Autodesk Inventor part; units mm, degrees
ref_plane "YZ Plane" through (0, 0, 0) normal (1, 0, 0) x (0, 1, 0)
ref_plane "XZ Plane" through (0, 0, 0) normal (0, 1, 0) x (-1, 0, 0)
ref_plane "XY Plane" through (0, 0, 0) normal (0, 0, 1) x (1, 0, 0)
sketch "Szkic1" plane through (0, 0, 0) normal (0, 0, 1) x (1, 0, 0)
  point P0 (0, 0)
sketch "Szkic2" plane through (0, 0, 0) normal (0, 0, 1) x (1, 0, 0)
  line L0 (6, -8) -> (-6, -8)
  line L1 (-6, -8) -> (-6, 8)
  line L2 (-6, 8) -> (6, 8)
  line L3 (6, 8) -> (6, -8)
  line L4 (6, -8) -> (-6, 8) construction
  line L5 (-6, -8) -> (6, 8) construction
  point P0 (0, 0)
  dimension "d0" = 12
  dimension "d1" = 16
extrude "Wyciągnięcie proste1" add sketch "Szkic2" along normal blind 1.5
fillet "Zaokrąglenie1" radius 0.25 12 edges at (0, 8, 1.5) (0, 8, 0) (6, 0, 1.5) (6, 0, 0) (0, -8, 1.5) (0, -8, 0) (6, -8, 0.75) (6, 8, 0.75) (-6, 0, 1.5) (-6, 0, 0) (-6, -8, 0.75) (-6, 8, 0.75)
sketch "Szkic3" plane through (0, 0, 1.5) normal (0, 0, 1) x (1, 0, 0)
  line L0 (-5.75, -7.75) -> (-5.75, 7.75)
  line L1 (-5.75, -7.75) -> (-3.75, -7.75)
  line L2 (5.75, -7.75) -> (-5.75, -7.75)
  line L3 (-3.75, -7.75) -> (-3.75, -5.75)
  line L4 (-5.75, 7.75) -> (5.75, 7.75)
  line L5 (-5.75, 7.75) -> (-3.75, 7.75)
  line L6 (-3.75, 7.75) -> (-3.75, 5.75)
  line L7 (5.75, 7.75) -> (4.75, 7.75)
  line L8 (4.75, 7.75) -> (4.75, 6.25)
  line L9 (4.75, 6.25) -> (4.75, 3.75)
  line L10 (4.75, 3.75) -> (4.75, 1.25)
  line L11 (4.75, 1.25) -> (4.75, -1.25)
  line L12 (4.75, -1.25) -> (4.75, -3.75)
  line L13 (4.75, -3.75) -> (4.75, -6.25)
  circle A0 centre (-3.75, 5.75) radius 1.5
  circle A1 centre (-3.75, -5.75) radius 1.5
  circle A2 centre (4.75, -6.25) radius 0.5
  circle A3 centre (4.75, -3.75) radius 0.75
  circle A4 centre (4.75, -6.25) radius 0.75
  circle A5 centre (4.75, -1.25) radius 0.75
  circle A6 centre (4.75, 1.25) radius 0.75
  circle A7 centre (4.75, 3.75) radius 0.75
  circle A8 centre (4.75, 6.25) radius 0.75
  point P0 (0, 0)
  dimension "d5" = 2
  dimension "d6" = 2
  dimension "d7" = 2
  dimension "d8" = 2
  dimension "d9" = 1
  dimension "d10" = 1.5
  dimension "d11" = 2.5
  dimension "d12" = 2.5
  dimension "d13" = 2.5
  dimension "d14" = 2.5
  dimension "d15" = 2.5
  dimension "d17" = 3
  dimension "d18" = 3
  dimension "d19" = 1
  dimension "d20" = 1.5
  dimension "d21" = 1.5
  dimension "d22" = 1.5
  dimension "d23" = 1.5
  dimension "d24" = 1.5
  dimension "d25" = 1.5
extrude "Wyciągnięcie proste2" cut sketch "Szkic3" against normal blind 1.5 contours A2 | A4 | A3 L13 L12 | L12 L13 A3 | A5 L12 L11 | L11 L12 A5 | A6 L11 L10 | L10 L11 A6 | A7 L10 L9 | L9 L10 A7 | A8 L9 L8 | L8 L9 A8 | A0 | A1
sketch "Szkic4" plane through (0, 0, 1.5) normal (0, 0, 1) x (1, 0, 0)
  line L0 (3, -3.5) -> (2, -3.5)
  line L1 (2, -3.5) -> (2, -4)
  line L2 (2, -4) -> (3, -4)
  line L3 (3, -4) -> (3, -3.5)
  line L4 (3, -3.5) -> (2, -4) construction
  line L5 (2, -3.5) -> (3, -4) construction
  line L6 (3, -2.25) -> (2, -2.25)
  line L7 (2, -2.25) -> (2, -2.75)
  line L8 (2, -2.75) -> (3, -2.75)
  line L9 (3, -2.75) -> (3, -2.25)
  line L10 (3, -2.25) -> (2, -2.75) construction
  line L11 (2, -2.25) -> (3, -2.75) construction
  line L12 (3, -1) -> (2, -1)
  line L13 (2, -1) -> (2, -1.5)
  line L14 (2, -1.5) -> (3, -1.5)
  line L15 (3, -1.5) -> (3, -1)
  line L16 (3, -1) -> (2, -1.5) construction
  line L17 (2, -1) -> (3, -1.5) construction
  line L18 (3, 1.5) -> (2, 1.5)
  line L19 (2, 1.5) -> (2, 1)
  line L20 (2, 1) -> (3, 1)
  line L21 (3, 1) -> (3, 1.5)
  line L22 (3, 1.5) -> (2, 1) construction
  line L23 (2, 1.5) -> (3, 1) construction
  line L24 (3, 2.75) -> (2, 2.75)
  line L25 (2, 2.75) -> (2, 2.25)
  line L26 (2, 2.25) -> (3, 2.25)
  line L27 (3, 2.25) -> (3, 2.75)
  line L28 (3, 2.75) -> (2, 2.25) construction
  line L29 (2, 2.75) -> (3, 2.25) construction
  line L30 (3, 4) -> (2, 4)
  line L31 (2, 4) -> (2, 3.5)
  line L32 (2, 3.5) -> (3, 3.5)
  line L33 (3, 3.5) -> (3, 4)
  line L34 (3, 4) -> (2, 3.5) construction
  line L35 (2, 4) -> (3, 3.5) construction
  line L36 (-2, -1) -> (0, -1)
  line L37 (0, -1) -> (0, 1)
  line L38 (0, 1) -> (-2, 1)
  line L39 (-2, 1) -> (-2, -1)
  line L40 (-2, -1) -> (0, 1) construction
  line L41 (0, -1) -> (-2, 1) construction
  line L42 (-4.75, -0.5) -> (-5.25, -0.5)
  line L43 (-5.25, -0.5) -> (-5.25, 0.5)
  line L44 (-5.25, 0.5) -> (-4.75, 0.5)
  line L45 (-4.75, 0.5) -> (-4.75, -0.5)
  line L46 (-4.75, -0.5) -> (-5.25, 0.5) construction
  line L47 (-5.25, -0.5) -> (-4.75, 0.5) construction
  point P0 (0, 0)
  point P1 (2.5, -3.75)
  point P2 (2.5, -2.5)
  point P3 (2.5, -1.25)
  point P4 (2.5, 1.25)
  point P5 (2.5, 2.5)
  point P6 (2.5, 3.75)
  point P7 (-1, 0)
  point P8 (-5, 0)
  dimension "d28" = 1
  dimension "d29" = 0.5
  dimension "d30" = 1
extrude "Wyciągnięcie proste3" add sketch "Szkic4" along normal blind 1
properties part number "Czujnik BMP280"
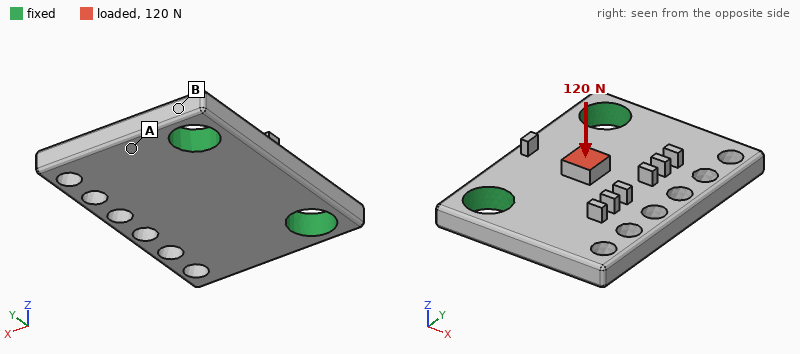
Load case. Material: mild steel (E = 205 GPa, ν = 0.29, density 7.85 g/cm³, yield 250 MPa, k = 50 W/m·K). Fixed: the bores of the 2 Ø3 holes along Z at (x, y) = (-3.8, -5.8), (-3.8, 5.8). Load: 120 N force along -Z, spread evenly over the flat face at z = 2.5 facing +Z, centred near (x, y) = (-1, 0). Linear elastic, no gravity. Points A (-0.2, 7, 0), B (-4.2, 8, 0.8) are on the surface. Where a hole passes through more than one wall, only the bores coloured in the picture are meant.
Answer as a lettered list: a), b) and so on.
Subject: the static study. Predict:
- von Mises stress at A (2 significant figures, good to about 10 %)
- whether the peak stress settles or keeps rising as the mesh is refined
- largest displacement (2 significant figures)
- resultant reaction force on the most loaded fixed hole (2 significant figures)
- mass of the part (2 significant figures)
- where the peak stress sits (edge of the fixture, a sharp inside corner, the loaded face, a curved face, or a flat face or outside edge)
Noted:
a) 22 MPa
b) keeps rising
c) 5.5 µm
d) 60 N
e) 2.0 g
f) edge of the fixture
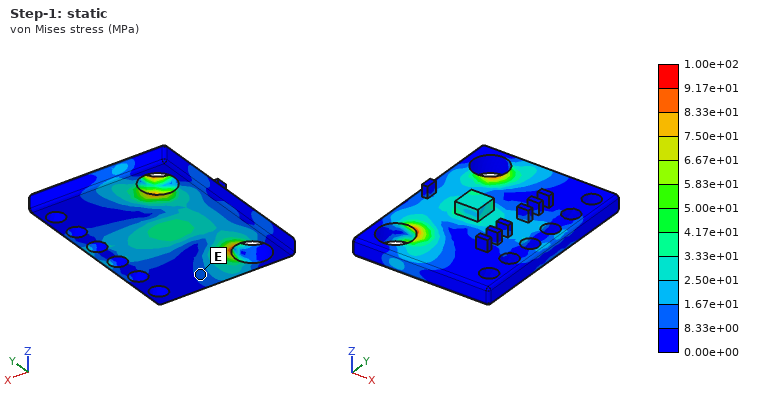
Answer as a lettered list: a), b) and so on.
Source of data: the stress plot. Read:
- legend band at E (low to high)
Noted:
a) 8.33e+00 to 1.67e+01 MPa
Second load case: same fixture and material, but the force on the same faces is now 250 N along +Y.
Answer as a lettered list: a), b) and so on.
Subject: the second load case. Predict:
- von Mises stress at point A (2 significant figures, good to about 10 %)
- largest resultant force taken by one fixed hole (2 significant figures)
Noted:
a) 6.7 MPa
b) 140 N
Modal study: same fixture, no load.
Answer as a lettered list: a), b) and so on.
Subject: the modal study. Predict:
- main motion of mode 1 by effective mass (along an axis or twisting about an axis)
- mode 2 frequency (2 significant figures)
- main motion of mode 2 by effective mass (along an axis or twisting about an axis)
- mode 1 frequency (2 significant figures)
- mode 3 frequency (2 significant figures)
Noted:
a) along Z
b) 27 kHz
c) twisting about X
d) 16 kHz
e) 45 kHz
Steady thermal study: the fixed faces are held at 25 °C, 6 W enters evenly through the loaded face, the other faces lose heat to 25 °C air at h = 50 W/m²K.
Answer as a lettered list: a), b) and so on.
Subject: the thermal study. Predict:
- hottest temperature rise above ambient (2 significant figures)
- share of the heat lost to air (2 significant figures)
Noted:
a) 70 K
b) 5.1 %
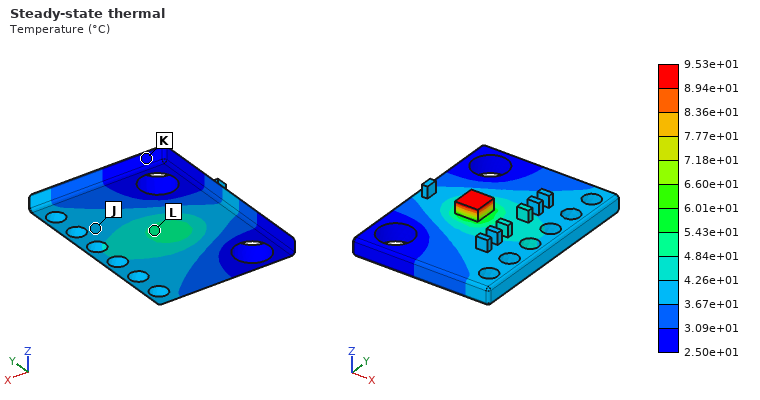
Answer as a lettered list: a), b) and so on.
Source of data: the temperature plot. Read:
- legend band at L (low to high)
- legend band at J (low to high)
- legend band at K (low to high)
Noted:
a) 4.84e+01 to 5.43e+01 °C
b) 3.67e+01 to 4.26e+01 °C
c) 2.50e+01 to 3.09e+01 °C
